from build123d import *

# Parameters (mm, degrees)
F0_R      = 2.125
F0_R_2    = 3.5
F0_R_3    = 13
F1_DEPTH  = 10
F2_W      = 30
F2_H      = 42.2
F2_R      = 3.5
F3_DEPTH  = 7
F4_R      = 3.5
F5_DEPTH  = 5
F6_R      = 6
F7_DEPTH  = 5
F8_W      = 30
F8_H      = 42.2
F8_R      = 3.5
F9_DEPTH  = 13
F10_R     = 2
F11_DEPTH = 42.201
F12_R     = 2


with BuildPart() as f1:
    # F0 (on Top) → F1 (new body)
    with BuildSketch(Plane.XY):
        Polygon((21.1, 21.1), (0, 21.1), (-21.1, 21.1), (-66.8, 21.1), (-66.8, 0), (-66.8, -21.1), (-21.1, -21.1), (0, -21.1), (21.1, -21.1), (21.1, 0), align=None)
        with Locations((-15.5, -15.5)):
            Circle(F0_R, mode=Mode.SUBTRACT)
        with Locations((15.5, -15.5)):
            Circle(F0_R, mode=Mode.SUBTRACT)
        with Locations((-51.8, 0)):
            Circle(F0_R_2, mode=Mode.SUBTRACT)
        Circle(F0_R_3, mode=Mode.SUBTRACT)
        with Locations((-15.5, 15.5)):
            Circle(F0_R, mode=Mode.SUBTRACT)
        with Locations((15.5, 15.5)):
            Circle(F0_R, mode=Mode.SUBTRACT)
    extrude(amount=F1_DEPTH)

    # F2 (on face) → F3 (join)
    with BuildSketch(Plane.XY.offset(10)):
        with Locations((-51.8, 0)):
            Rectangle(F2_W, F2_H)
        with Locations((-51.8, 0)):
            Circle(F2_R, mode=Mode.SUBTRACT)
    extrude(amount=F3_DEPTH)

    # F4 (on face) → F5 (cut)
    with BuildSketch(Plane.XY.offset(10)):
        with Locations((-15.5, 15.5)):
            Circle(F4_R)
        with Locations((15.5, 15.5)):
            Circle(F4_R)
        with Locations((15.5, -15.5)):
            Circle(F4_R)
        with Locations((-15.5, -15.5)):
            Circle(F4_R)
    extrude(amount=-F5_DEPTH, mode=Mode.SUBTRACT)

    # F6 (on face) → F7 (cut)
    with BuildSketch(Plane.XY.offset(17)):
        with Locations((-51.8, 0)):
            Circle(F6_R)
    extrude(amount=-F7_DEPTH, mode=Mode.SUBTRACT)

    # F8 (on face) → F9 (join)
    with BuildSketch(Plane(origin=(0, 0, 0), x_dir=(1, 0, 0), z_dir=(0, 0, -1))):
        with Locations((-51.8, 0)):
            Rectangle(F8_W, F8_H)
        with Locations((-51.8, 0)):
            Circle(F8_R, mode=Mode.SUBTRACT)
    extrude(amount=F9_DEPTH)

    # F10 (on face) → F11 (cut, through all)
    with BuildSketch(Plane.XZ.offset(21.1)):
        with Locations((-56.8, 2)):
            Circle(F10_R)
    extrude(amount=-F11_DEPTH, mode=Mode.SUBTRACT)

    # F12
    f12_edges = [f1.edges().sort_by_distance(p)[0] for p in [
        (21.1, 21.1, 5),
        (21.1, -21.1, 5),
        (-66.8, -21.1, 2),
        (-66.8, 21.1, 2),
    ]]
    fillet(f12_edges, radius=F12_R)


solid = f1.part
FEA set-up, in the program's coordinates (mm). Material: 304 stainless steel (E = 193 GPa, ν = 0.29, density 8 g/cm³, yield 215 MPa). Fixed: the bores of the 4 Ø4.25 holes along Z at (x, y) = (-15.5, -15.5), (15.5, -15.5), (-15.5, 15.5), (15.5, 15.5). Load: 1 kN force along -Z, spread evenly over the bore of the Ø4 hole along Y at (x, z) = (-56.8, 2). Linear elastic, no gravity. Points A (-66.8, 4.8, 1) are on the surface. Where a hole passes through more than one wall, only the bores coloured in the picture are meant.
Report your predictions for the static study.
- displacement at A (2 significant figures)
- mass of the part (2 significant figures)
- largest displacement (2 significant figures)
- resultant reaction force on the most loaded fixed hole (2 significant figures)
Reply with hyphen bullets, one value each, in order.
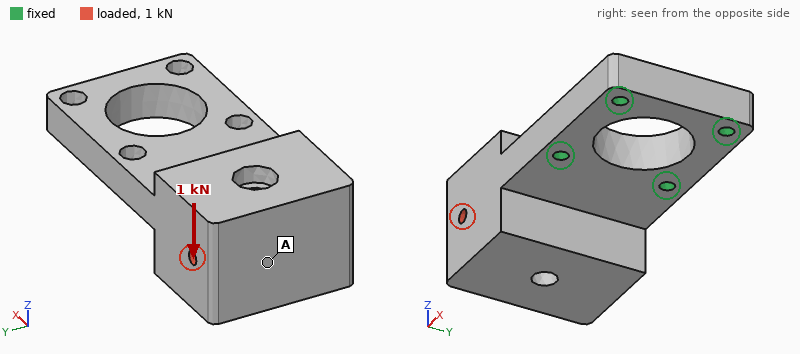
- 80 µm
- 430 g
- 86 µm
- 1.0 kN
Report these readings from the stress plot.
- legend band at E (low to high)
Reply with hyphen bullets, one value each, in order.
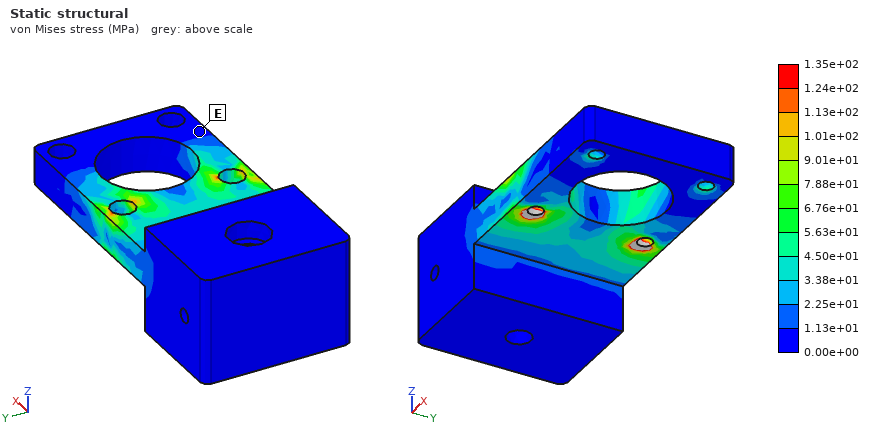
- 0.00e+00 to 1.13e+01 MPa
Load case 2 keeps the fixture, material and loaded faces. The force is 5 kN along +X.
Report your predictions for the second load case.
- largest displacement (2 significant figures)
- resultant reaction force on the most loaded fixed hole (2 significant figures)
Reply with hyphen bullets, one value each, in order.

- 26 µm
- 2.5 kN
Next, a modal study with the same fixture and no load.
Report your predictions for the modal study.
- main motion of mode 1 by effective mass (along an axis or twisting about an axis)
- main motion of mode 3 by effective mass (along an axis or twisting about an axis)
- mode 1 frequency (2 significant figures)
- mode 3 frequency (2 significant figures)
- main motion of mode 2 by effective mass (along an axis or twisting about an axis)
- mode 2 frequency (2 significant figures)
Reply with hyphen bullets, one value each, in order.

- along Z
- along Y
- 1300 Hz
- 5800 Hz
- along Y
- 4300 Hz
